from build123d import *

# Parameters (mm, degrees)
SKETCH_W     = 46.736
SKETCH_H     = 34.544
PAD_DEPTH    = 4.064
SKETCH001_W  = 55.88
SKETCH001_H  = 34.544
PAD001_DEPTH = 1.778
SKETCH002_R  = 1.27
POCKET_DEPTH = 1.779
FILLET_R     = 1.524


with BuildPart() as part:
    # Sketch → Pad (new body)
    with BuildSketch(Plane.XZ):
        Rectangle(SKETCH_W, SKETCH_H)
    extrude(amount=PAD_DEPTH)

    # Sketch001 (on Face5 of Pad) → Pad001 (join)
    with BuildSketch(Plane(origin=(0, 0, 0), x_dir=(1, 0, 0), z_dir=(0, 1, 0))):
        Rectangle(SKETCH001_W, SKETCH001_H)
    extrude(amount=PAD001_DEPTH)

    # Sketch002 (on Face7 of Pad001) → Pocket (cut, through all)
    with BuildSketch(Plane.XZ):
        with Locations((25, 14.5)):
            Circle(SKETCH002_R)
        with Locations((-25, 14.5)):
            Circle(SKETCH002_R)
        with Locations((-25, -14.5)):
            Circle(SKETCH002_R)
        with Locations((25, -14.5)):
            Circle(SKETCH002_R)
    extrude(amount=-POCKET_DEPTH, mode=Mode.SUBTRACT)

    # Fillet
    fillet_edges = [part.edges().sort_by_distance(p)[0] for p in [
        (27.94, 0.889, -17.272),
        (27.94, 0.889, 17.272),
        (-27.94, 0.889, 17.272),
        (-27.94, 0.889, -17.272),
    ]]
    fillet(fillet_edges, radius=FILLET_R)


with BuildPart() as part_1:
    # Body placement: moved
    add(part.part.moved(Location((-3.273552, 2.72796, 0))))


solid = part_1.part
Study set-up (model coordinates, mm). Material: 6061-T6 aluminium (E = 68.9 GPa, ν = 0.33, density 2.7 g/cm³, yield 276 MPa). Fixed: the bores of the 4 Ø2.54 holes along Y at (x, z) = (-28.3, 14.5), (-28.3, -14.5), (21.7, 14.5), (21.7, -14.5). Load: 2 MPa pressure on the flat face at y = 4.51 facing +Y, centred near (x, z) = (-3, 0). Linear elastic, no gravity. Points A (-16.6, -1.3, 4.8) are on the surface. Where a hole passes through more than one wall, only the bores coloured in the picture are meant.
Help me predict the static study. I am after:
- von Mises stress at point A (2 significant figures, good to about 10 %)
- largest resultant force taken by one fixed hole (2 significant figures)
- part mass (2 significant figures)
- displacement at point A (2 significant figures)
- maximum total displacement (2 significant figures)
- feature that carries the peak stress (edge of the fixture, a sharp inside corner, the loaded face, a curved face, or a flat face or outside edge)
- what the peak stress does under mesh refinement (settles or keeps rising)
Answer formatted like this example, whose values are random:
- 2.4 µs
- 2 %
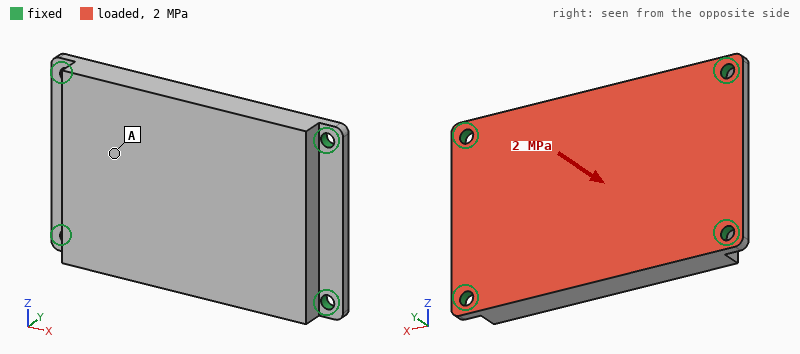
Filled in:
- 41 MPa
- 1.6 kN
- 27 g
- 60 µm
- 85 µm
- edge of the fixture
- keeps rising
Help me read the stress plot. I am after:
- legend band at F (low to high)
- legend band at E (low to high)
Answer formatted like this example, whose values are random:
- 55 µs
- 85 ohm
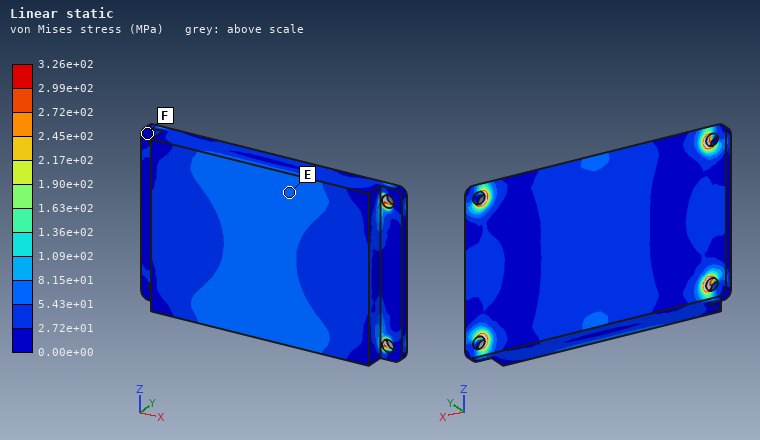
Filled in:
- 0.00e+00 to 2.72e+01 MPa
- 5.43e+01 to 8.15e+01 MPa
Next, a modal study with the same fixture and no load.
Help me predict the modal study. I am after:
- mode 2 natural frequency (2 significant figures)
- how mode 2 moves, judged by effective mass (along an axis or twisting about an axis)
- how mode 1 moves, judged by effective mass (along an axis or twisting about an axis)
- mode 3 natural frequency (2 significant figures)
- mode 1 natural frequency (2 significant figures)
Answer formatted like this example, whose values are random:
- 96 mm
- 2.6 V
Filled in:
- 12 kHz
- twisting about X
- along Y
- 16 kHz
- 6900 Hz
